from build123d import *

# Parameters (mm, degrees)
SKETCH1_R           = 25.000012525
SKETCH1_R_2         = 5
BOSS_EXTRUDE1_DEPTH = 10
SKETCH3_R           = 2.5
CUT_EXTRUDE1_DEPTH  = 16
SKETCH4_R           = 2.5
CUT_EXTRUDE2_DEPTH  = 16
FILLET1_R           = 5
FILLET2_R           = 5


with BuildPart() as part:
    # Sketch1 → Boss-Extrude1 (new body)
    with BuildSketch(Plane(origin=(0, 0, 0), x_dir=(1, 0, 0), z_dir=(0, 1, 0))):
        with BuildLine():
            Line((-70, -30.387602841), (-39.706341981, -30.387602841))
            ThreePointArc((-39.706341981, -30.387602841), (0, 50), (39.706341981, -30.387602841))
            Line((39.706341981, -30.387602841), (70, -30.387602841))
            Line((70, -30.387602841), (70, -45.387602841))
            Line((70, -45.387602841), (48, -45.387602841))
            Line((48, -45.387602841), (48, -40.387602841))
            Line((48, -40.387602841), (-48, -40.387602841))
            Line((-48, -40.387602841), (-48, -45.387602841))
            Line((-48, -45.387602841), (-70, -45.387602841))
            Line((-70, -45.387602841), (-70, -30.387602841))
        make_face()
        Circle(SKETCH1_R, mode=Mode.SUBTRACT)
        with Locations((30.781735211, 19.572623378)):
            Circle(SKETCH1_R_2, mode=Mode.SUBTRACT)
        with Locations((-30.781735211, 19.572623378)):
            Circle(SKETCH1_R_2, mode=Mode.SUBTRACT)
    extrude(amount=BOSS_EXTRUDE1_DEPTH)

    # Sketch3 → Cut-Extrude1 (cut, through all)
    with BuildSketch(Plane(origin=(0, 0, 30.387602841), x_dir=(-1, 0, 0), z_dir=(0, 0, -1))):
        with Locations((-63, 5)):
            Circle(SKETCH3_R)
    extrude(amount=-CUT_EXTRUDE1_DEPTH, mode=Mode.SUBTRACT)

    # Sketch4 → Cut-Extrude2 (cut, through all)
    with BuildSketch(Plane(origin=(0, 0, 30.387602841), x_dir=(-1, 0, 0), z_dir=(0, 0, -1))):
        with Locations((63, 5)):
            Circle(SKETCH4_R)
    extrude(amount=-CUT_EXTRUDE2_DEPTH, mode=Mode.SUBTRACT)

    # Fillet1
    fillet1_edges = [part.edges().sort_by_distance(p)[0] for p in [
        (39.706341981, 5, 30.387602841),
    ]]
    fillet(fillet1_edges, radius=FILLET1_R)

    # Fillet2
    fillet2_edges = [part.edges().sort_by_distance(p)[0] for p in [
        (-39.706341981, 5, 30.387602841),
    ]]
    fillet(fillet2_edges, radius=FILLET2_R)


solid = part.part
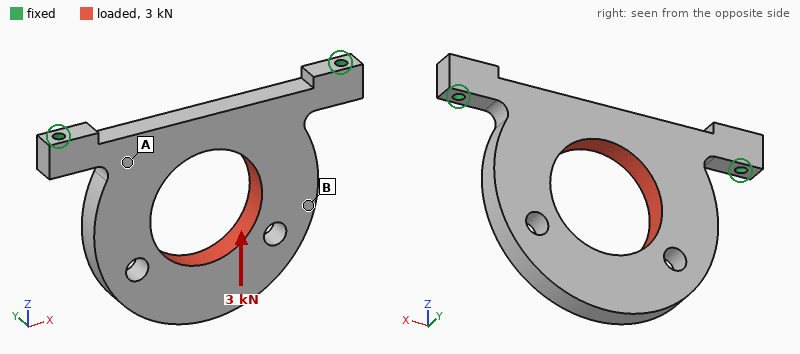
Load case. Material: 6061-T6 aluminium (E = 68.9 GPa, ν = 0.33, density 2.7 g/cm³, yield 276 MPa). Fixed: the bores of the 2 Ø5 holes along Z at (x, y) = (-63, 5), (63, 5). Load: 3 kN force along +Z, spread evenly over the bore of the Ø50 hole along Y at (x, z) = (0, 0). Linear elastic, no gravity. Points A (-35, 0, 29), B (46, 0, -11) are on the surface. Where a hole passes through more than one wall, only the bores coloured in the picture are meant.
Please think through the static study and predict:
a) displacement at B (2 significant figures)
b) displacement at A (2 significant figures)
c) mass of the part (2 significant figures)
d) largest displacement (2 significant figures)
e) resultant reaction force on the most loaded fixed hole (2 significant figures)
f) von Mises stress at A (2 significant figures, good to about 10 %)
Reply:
27 µm
24 µm
170 g
34 µm
1.8 kN
9.2 MPa
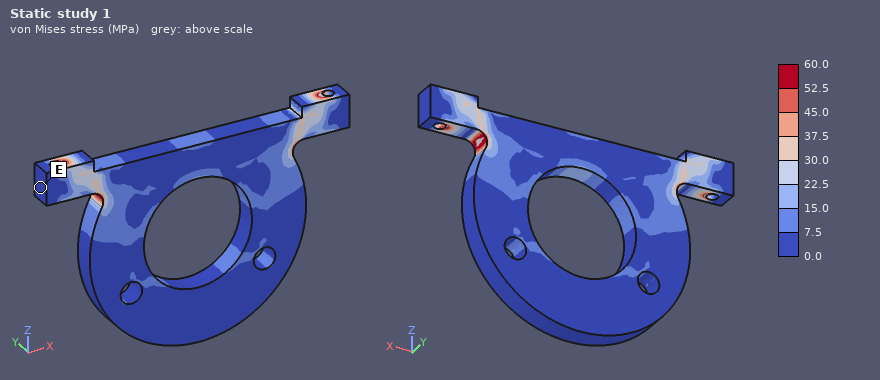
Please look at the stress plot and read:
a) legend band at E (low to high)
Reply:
0.0 to 7.5 MPa
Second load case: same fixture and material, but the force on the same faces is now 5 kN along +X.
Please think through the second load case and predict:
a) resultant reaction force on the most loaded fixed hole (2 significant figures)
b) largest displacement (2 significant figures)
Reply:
3.1 kN
76 µm
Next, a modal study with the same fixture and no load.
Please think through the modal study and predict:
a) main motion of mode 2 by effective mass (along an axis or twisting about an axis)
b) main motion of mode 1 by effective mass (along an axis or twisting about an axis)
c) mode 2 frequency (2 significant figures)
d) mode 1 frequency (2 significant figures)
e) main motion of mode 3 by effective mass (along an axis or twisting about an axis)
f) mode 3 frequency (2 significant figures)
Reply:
twisting about Z
along Y
2000 Hz
540 Hz
along Y
2900 Hz
